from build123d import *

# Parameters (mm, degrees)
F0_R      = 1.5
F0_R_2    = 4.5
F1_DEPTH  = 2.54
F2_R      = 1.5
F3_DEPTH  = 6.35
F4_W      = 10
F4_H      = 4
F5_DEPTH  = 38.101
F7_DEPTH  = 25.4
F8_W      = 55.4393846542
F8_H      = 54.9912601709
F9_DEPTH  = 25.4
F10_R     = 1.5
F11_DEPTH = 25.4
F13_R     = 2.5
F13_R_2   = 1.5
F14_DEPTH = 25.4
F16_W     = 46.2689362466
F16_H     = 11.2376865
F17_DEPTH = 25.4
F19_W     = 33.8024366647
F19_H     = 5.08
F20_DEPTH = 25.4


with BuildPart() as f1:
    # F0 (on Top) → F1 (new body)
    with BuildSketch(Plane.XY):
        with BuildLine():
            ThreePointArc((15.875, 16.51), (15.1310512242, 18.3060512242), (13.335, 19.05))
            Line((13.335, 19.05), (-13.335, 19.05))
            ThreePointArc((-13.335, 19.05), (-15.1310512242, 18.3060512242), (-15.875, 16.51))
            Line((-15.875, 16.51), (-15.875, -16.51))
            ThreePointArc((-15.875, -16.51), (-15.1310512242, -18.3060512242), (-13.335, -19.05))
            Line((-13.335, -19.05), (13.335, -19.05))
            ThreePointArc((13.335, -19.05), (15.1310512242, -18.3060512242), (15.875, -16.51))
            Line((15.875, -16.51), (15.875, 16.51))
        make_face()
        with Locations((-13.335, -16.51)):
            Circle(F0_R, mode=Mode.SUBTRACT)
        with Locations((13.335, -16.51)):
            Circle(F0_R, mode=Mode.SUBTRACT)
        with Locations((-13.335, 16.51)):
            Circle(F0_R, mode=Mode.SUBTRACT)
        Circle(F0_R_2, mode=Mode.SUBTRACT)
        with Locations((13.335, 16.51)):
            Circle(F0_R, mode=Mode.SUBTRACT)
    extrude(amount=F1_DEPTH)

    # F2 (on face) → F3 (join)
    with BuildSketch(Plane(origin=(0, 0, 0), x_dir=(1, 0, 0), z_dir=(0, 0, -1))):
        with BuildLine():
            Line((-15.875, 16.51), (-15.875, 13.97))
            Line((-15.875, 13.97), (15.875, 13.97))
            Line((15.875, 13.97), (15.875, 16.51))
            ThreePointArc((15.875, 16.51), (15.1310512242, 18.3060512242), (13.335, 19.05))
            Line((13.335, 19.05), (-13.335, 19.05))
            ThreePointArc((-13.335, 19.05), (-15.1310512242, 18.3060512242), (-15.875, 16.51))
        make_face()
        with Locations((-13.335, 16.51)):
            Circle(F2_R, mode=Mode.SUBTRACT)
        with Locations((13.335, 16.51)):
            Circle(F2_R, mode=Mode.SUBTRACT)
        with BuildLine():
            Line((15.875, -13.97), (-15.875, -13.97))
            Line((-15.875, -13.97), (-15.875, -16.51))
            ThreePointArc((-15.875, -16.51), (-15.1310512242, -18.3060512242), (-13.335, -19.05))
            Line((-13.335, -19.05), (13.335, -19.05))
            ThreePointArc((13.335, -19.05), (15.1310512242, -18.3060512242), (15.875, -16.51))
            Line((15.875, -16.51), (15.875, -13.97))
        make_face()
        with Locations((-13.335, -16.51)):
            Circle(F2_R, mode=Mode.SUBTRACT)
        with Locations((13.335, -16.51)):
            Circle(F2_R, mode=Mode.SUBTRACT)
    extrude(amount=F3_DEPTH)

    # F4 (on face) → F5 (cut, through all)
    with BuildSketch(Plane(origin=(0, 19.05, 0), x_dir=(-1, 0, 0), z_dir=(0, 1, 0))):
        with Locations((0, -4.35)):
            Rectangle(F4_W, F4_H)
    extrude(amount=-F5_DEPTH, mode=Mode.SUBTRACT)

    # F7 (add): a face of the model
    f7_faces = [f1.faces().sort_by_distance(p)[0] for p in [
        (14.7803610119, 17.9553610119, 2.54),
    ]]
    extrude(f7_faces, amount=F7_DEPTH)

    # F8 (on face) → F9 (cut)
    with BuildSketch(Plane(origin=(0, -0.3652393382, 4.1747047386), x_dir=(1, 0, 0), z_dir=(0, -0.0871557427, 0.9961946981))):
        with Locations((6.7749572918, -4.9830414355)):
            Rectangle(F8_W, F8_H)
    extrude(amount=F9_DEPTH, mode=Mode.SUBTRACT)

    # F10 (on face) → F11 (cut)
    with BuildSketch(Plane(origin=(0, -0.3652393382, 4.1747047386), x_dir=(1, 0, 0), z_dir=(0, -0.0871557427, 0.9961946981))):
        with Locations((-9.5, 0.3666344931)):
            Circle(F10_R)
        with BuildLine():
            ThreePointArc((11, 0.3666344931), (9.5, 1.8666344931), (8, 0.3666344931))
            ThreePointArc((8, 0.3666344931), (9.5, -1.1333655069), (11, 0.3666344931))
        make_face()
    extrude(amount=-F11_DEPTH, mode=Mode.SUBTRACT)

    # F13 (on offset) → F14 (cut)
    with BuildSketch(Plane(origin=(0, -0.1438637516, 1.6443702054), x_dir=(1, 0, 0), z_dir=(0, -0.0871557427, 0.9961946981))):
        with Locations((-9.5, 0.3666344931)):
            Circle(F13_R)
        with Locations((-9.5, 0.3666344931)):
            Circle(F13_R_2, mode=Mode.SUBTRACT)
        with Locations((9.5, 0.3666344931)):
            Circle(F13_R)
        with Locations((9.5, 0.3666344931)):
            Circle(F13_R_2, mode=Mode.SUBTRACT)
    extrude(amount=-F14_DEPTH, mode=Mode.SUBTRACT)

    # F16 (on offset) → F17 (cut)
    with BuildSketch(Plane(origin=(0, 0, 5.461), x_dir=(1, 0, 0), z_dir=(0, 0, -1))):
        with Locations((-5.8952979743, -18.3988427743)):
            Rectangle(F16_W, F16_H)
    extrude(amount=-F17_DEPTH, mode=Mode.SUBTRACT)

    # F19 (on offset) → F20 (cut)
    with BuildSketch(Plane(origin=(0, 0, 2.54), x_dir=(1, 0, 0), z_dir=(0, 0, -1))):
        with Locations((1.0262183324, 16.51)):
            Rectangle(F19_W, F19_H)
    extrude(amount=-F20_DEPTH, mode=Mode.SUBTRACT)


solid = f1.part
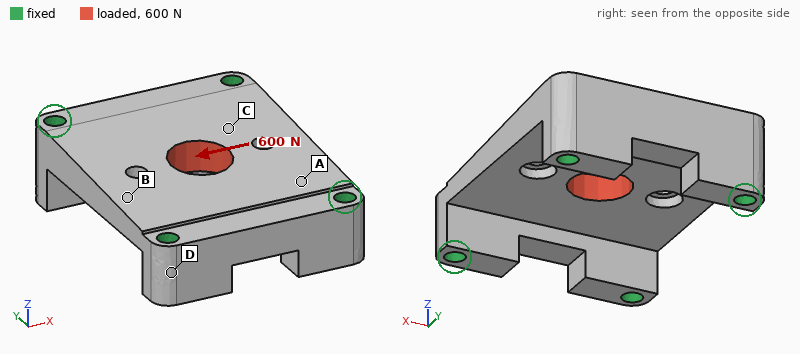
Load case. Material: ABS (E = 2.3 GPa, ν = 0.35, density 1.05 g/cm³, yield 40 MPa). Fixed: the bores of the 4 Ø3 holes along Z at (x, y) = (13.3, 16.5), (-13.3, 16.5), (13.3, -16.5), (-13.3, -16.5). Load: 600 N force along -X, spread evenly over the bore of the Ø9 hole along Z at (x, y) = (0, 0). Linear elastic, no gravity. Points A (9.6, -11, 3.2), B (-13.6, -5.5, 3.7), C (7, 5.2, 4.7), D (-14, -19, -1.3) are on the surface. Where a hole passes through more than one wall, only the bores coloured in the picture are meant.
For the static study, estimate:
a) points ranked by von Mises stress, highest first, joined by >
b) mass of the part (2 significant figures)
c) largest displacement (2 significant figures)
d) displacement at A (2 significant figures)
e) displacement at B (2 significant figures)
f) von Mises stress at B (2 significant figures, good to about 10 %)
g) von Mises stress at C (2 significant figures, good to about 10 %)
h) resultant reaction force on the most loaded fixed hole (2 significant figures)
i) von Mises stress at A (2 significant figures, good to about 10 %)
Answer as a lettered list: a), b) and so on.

a) A > C > B > D
b) 6.2 g
c) 60 µm
d) 22 µm
e) 39 µm
f) 2.7 MPa
g) 3.9 MPa
h) 210 N
i) 5.2 MPa
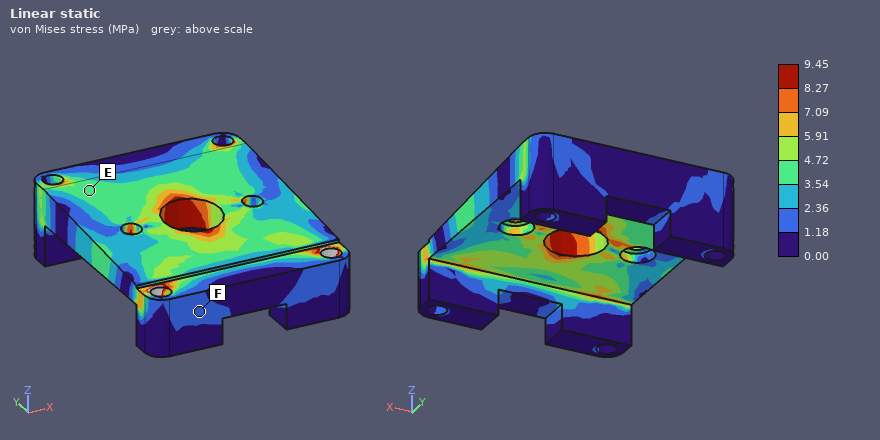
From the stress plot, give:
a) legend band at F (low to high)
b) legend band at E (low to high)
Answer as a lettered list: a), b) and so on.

a) 1.18 to 2.36 MPa
b) 3.54 to 4.72 MPa
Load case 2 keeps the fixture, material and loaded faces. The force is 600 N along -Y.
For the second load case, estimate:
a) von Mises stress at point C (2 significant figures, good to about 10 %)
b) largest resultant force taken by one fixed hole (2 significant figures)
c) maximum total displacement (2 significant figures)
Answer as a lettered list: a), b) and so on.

a) 2.8 MPa
b) 200 N
c) 60 µm
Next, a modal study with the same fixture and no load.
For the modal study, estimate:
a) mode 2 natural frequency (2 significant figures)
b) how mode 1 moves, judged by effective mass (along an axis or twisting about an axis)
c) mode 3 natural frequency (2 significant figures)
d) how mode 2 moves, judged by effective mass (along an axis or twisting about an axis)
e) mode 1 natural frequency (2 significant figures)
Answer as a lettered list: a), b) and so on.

a) 6800 Hz
b) along Z
c) 9700 Hz
d) twisting about Y
e) 5200 Hz
